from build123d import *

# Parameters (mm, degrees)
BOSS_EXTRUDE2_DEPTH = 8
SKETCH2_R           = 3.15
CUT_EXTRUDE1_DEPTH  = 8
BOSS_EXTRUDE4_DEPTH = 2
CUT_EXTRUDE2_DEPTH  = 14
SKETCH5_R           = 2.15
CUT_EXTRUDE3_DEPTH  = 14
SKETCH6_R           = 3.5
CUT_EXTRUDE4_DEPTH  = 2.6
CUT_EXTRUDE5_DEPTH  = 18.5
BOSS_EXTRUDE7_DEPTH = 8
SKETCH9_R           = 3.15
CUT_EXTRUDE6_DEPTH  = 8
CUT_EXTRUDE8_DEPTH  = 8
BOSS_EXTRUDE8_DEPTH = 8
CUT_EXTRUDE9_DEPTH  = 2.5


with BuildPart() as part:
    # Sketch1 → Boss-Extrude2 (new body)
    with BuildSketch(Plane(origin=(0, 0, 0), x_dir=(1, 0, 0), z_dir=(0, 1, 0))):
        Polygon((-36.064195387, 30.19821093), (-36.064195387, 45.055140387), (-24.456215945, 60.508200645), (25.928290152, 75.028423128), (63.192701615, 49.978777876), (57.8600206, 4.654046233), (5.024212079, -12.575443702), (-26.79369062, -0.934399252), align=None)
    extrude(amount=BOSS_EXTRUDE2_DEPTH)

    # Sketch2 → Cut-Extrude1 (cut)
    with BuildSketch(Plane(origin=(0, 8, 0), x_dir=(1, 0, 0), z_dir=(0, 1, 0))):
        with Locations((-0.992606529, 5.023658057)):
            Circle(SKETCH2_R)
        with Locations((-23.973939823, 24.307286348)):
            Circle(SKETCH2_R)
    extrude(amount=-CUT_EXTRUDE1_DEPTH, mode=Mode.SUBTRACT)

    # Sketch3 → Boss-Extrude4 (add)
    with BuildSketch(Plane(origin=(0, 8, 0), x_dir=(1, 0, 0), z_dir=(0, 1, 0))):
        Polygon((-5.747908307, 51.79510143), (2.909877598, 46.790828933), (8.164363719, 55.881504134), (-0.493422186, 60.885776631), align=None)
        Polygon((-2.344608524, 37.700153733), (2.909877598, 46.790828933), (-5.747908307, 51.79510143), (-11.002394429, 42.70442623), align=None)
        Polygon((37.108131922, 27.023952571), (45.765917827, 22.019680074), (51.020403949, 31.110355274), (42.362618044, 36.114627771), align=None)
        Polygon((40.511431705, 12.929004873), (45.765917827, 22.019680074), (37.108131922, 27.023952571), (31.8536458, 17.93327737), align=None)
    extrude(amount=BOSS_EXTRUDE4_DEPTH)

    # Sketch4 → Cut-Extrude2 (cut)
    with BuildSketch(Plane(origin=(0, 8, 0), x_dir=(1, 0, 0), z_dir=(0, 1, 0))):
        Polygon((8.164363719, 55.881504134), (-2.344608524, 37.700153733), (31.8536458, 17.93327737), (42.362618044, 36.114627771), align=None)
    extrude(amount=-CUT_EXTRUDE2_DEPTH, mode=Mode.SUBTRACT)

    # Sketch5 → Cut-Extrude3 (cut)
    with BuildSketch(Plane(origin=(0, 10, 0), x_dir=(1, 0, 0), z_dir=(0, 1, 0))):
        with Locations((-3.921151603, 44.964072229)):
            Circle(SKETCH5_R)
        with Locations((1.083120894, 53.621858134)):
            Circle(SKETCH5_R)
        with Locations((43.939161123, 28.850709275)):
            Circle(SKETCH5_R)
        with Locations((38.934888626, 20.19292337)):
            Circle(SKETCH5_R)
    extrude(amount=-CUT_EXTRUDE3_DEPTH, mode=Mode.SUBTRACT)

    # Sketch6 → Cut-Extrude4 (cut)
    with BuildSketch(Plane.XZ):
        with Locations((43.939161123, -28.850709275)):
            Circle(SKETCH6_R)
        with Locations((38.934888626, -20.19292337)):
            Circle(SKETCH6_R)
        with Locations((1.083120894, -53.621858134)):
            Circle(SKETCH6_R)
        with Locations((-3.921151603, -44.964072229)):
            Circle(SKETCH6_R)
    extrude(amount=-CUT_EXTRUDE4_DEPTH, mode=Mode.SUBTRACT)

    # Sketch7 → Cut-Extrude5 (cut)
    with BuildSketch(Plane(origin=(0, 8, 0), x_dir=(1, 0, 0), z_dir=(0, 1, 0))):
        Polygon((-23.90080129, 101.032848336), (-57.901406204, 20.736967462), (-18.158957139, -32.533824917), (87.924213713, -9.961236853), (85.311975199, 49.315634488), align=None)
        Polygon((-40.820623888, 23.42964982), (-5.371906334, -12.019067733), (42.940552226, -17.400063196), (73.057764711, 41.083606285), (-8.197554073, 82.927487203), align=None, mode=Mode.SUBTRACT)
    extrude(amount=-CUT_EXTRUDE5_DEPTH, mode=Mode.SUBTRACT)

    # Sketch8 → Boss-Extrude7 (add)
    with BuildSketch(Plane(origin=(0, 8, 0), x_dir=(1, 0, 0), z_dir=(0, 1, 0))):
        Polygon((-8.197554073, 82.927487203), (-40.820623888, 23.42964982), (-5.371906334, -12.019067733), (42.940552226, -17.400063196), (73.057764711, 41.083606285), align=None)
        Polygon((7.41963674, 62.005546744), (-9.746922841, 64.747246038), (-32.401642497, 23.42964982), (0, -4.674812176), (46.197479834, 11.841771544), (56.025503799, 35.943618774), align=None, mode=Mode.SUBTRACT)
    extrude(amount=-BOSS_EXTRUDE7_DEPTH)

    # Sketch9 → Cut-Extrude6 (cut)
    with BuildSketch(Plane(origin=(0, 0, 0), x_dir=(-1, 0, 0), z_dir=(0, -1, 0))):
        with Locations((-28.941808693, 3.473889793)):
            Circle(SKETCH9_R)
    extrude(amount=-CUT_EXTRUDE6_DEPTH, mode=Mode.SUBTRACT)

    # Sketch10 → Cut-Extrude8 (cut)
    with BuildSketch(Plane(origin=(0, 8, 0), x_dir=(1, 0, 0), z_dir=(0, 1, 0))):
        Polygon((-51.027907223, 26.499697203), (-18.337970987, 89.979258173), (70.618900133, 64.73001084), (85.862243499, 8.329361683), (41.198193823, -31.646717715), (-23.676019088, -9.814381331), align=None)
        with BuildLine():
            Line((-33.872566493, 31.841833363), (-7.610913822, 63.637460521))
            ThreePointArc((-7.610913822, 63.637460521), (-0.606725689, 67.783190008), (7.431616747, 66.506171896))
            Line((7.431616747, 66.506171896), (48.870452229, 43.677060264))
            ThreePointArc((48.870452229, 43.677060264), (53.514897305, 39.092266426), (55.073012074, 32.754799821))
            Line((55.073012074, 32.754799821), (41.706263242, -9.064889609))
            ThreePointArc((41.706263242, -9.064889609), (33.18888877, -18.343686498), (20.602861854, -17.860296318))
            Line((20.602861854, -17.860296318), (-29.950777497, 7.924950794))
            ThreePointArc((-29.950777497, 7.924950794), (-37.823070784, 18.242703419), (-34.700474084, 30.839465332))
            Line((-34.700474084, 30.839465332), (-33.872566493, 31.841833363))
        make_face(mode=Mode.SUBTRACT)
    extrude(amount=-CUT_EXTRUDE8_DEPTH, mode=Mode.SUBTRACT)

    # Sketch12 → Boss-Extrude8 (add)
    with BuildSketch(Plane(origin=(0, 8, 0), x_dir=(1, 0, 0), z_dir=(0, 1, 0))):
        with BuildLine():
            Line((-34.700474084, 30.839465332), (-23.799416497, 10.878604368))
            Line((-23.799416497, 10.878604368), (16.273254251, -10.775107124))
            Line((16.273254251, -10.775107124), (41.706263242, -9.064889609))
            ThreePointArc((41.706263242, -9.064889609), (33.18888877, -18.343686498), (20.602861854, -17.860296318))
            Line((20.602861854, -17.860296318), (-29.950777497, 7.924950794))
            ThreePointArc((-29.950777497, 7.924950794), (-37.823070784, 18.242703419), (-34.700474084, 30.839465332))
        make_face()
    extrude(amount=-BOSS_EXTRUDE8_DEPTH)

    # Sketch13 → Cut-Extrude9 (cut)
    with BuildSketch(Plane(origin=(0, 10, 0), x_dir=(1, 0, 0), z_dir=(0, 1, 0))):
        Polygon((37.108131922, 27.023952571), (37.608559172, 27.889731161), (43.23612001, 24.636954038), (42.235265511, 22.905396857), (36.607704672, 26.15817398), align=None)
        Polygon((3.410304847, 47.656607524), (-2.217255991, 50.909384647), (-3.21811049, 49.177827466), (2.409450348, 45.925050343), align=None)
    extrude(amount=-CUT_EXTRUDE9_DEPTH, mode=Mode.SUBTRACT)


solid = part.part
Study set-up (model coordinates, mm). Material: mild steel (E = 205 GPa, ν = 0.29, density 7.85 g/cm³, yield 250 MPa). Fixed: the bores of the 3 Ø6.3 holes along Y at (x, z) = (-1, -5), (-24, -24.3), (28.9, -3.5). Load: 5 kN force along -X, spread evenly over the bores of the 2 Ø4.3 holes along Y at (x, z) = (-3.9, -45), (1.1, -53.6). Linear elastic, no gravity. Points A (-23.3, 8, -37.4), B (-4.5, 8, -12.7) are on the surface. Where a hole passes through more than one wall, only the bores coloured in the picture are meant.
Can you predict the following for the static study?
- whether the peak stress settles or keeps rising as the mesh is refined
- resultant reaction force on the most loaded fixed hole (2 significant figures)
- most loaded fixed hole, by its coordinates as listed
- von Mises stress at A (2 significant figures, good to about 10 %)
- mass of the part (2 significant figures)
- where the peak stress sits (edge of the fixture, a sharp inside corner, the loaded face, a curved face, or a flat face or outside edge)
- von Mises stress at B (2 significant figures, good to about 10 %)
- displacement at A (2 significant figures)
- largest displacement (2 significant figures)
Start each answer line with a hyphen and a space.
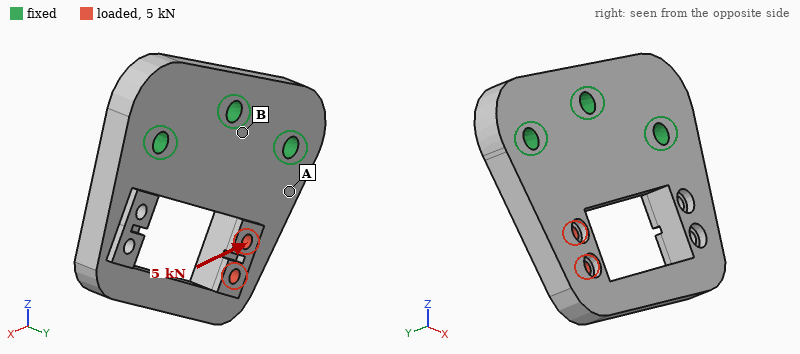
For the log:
- keeps rising
- 5.0 kN
- (-24, -24.3)
- 43 MPa
- 270 g
- a sharp inside corner
- 14 MPa
- 4.5 µm
- 23 µm
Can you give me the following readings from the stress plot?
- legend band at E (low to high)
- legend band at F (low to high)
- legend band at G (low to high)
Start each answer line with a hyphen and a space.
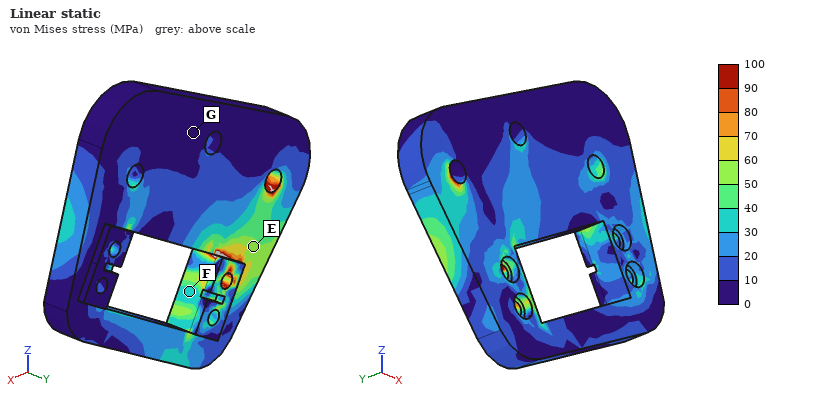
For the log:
- 50 to 60 MPa
- 30 to 40 MPa
- 0 to 10 MPa
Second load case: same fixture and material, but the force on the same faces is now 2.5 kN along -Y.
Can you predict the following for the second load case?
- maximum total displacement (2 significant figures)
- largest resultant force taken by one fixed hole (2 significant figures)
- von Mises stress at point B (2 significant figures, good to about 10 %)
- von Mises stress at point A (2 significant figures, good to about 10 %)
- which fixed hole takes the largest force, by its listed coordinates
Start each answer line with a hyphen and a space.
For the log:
- 0.15 mm
- 2.1 kN
- 50 MPa
- 120 MPa
- (-24, -24.3)
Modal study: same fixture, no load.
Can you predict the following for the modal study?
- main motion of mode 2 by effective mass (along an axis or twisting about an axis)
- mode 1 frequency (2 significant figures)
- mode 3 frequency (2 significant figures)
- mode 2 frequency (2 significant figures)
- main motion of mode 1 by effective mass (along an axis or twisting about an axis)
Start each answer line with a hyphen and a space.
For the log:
- twisting about Z
- 2700 Hz
- 7900 Hz
- 4700 Hz
- along Y
